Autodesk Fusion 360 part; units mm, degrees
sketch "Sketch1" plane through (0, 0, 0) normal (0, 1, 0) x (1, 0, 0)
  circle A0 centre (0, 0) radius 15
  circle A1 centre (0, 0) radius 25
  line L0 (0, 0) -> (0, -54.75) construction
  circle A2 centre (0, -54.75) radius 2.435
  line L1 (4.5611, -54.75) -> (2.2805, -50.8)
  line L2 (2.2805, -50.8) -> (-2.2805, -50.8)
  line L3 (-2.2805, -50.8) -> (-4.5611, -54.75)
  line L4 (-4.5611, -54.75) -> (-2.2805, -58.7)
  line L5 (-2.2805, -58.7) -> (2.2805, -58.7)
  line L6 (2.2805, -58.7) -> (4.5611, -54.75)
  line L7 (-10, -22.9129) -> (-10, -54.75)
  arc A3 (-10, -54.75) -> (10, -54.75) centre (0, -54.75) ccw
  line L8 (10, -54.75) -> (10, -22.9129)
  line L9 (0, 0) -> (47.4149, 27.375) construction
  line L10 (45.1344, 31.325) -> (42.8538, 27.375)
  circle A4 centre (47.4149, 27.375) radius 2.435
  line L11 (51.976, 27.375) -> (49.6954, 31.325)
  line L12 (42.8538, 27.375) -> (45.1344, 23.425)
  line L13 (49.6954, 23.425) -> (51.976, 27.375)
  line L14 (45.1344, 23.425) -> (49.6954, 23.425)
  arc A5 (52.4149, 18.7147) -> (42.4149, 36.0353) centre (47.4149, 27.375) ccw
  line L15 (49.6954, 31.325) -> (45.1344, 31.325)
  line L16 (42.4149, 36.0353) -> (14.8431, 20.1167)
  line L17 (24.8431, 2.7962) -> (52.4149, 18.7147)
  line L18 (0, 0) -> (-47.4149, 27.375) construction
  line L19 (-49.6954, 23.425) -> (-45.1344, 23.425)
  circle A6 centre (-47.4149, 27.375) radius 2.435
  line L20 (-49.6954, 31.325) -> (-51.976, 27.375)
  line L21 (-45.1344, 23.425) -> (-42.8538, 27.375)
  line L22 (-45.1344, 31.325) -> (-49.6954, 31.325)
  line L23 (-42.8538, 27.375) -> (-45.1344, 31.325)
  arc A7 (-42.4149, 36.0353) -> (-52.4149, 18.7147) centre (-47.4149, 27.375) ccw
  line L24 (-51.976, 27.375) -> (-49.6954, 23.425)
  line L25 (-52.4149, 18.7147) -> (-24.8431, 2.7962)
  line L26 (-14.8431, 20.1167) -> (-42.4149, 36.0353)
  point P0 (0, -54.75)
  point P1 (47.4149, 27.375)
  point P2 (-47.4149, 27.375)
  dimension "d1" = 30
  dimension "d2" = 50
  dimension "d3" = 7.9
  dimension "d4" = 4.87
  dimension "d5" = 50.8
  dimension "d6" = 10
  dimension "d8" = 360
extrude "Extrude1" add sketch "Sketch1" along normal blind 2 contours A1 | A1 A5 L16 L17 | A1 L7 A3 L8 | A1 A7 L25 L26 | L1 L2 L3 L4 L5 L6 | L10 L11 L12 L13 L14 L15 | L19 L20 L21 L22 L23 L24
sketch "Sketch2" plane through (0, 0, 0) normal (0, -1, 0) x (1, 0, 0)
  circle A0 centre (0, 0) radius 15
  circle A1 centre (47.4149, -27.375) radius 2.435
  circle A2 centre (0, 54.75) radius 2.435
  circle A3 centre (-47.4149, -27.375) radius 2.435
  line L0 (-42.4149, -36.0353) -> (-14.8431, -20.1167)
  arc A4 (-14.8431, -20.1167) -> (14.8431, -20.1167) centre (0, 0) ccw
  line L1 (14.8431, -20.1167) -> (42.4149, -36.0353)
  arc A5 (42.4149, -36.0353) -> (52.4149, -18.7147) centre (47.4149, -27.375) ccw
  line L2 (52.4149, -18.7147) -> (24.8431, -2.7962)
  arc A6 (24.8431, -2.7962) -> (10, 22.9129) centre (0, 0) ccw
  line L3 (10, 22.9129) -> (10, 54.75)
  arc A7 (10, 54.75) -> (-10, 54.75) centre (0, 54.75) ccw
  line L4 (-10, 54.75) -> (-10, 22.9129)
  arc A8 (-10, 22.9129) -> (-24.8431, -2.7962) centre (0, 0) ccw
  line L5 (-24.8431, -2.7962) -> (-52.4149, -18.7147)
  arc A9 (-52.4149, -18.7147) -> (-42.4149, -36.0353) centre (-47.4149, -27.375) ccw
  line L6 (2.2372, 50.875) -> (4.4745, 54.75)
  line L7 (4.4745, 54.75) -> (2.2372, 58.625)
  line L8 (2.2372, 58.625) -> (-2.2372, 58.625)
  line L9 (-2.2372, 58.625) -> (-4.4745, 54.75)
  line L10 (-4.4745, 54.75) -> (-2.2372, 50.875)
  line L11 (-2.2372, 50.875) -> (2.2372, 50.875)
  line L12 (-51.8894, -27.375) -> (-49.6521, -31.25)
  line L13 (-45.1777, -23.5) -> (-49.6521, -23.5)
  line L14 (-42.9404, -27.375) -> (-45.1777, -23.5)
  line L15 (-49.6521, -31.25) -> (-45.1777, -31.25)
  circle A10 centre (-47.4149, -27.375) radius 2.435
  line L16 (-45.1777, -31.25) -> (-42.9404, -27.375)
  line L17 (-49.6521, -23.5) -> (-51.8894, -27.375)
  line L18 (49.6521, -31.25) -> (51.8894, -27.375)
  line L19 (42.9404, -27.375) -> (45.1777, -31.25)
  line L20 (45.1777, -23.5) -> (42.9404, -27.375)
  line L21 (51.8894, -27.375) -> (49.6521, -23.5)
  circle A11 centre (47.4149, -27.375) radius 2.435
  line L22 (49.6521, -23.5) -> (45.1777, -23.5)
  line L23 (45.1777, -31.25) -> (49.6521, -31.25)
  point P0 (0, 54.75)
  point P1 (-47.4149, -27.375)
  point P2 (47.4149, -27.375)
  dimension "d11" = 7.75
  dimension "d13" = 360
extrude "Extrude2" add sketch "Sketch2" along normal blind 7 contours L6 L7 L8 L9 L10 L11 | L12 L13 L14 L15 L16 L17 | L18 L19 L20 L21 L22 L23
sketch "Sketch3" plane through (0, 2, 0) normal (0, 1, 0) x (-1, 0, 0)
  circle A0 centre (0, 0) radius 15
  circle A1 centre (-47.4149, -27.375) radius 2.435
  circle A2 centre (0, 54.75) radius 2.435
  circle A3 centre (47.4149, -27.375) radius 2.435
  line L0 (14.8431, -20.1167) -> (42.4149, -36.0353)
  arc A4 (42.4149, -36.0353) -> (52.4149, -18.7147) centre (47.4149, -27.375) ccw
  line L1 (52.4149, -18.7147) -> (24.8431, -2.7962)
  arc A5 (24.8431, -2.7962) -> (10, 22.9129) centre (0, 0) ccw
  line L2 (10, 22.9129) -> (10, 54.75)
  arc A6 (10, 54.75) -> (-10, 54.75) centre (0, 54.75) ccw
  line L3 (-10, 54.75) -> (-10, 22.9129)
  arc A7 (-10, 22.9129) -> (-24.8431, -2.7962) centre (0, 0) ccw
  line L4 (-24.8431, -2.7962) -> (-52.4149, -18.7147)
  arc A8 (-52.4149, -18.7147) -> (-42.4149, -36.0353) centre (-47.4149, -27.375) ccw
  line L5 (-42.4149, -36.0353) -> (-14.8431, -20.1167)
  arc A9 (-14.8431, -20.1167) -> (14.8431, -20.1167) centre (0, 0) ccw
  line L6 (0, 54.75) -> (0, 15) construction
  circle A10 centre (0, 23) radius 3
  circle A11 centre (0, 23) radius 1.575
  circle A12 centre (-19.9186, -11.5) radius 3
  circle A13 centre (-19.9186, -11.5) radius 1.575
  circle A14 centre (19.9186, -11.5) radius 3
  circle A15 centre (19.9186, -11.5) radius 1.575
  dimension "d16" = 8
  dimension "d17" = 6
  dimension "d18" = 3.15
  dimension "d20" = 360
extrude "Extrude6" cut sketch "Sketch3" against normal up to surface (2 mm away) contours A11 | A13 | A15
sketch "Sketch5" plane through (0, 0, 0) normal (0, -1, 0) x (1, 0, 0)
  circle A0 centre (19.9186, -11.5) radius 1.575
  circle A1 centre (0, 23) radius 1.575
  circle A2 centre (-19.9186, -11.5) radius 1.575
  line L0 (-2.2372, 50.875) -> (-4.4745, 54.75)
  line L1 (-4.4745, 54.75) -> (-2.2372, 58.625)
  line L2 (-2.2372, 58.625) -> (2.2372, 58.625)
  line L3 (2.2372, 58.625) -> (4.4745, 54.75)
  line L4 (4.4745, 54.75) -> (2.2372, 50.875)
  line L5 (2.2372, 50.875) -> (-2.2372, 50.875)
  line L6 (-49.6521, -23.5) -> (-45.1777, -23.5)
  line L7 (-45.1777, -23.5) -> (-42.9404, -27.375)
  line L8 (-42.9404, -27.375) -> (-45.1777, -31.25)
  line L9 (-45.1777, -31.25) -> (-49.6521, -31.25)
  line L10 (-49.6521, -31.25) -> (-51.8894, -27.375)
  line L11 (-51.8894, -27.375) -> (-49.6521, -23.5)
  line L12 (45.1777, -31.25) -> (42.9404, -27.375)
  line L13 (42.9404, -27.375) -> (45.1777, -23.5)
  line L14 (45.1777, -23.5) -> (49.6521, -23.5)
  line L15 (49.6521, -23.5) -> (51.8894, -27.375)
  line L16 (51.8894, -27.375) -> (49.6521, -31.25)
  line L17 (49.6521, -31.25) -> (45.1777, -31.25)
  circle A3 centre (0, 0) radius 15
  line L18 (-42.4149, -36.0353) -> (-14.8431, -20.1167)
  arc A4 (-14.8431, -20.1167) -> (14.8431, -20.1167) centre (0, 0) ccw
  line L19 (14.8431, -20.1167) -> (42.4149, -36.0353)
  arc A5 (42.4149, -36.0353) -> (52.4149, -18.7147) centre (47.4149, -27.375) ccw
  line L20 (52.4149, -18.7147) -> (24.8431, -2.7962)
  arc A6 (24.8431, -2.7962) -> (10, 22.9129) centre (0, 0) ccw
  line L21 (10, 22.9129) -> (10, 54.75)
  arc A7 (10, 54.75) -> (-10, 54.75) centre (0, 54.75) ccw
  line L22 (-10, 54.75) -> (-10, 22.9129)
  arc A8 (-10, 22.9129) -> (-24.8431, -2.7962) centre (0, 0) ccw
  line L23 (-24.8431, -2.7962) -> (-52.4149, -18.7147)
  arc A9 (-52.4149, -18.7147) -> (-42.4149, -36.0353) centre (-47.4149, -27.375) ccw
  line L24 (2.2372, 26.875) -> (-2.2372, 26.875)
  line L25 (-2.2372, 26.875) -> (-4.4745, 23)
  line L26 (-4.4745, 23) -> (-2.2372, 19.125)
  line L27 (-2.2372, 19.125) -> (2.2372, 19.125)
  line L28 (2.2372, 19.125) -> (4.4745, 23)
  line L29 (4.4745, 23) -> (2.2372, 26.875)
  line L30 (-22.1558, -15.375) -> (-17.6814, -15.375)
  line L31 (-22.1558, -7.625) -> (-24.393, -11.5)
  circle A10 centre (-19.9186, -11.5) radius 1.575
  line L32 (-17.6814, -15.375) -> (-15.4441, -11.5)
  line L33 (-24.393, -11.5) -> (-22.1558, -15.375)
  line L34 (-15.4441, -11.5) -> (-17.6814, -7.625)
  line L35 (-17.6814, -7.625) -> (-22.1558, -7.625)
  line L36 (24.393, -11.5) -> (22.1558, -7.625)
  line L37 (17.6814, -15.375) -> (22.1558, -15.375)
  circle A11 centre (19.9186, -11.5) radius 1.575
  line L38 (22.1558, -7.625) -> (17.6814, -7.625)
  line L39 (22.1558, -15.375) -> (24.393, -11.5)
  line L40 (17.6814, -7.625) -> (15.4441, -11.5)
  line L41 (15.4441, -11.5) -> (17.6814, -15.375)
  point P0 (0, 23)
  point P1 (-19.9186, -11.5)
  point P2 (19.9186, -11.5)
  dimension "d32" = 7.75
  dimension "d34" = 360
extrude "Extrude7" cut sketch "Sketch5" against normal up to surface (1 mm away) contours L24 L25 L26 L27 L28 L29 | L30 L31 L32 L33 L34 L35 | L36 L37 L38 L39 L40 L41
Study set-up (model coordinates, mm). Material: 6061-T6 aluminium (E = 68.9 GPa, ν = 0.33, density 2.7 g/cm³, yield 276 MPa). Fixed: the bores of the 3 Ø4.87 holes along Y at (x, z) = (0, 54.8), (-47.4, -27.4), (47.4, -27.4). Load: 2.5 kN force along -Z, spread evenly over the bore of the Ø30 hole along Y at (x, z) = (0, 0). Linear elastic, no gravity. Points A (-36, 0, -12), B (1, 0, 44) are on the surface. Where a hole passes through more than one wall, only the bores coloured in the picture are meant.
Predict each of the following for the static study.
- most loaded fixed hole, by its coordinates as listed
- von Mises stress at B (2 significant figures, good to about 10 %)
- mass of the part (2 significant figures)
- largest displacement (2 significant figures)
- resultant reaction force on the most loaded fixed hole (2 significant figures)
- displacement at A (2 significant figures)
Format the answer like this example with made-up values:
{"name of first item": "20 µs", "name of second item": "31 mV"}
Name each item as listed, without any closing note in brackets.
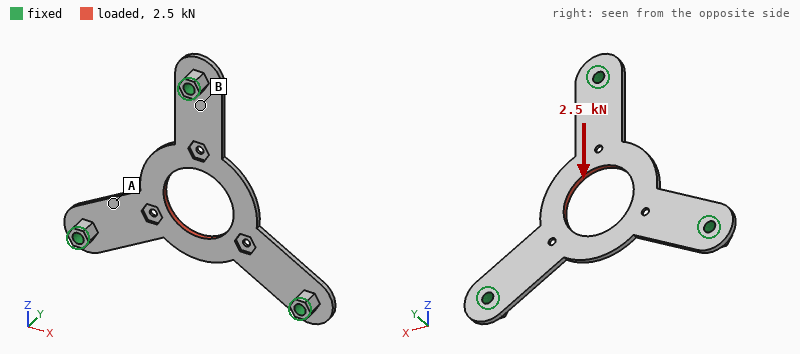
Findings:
{"most loaded fixed hole, by its coordinates as listed": "(0, 54.8)", "von Mises stress at B": "46 MPa", "mass of the part": "20 g", "largest displacement": "0.10 mm", "resultant reaction force on the most loaded fixed hole": "1.5 kN", "displacement at A": "0.029 mm"}
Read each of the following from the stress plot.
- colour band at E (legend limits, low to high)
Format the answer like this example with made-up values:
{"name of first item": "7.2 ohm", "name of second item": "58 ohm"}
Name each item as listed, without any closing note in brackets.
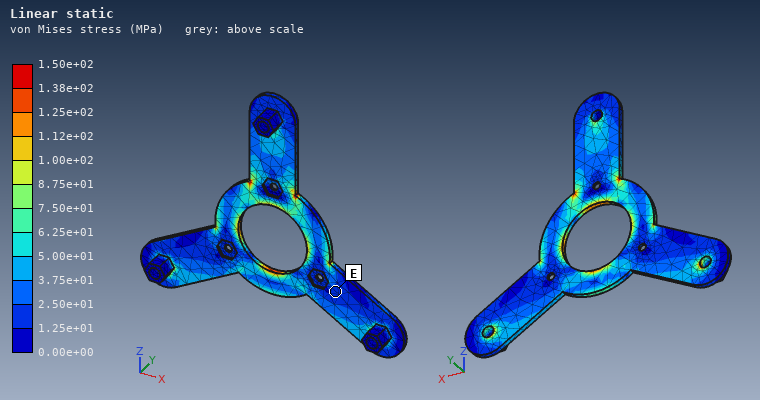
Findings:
{"colour band at E": "1.25e+01 to 2.50e+01 MPa"}
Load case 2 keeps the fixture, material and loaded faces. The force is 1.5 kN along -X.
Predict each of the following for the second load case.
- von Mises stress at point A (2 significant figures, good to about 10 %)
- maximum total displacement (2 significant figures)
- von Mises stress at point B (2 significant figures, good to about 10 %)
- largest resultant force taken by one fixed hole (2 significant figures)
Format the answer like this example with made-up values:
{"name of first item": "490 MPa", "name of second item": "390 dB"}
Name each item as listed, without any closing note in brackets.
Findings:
{"von Mises stress at point A": "25 MPa", "maximum total displacement": "57 µm", "von Mises stress at point B": "9.0 MPa", "largest resultant force taken by one fixed hole": "760 N"}
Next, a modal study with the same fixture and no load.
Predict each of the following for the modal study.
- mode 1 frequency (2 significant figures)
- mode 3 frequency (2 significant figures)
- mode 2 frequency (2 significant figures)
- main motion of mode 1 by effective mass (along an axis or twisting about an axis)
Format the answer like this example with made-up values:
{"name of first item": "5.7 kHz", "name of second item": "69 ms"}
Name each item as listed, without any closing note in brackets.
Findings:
{"mode 1 frequency": "1100 Hz", "mode 3 frequency": "2100 Hz", "mode 2 frequency": "2100 Hz", "main motion of mode 1 by effective mass": "along Y"}
